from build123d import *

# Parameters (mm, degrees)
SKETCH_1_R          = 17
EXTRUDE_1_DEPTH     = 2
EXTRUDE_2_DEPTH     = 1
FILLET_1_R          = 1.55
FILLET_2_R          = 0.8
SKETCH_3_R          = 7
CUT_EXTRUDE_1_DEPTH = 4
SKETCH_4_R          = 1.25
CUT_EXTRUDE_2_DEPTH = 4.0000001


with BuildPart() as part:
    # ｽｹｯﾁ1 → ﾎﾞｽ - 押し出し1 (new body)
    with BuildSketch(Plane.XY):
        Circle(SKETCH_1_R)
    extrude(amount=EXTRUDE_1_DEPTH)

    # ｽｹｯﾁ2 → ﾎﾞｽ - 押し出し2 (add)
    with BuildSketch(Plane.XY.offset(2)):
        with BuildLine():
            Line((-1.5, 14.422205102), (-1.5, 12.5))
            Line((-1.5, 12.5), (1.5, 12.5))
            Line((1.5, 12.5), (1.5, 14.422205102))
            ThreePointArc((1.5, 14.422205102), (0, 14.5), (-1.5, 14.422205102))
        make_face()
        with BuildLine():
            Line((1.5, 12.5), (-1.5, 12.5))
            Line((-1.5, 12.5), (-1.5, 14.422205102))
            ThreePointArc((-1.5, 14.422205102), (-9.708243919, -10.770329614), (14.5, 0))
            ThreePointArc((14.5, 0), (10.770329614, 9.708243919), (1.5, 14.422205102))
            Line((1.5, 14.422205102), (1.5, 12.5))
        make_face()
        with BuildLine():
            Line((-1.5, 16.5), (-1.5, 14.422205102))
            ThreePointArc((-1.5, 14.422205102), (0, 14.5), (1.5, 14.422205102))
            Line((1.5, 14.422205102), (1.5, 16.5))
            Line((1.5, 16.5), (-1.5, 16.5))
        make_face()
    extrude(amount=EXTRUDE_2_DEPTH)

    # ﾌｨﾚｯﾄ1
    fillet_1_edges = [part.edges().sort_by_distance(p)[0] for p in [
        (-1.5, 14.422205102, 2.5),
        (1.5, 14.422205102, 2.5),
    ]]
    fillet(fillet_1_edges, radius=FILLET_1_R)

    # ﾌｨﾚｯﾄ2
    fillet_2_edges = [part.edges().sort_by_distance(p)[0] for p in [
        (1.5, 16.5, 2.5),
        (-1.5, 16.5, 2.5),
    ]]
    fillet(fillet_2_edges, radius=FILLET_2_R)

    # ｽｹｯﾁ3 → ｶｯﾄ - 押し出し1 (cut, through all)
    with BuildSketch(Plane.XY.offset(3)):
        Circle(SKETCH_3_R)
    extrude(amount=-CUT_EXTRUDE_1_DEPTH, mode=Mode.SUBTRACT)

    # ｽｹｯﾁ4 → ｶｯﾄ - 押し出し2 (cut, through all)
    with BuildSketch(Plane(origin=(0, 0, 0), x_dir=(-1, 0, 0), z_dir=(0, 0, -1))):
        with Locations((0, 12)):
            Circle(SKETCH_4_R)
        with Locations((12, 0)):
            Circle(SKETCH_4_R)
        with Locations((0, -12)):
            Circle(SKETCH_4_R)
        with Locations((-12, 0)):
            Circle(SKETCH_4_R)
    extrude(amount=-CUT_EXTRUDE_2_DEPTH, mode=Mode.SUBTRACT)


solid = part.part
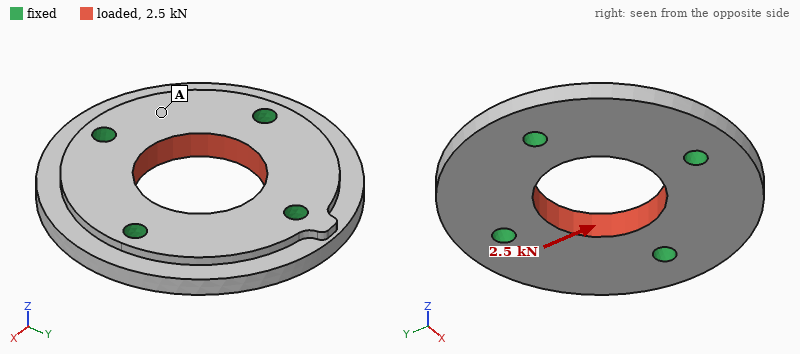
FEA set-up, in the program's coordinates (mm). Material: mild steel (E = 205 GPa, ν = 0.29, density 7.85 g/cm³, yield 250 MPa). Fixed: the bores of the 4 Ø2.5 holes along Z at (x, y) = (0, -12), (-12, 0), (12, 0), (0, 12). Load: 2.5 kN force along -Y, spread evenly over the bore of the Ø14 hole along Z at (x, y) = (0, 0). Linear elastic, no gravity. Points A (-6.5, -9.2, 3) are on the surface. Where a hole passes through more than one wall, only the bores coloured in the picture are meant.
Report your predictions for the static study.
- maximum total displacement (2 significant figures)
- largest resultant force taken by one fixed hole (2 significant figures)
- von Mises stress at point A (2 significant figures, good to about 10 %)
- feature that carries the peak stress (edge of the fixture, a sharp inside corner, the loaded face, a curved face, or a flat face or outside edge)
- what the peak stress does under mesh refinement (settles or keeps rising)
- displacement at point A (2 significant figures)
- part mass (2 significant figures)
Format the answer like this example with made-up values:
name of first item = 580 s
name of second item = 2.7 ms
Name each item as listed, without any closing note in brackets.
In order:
maximum total displacement = 1.2 µm
largest resultant force taken by one fixed hole = 650 N
von Mises stress at point A = 12 MPa
feature that carries the peak stress = edge of the fixture
what the peak stress does under mesh refinement = keeps rising
displacement at point A = 0.84 µm
part mass = 15 g
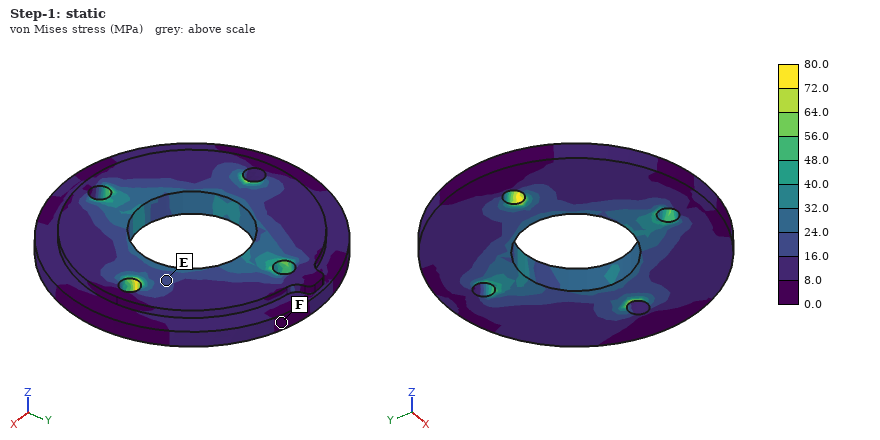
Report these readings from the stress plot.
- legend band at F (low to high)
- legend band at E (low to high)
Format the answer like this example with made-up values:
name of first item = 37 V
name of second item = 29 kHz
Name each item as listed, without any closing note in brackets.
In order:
legend band at F = 0.0 to 8.0 MPa
legend band at E = 16.0 to 24.0 MPa
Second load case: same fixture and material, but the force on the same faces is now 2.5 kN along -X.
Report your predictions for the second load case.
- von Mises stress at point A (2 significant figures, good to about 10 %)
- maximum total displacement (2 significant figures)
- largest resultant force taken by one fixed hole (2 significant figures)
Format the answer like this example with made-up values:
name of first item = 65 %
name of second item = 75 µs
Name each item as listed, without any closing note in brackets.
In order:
von Mises stress at point A = 11 MPa
maximum total displacement = 1.2 µm
largest resultant force taken by one fixed hole = 650 N
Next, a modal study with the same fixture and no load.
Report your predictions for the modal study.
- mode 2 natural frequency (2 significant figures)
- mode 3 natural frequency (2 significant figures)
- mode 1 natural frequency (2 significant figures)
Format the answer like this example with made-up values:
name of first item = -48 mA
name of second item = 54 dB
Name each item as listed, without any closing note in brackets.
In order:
mode 2 natural frequency = 31 kHz
mode 3 natural frequency = 31 kHz
mode 1 natural frequency = 30 kHz
